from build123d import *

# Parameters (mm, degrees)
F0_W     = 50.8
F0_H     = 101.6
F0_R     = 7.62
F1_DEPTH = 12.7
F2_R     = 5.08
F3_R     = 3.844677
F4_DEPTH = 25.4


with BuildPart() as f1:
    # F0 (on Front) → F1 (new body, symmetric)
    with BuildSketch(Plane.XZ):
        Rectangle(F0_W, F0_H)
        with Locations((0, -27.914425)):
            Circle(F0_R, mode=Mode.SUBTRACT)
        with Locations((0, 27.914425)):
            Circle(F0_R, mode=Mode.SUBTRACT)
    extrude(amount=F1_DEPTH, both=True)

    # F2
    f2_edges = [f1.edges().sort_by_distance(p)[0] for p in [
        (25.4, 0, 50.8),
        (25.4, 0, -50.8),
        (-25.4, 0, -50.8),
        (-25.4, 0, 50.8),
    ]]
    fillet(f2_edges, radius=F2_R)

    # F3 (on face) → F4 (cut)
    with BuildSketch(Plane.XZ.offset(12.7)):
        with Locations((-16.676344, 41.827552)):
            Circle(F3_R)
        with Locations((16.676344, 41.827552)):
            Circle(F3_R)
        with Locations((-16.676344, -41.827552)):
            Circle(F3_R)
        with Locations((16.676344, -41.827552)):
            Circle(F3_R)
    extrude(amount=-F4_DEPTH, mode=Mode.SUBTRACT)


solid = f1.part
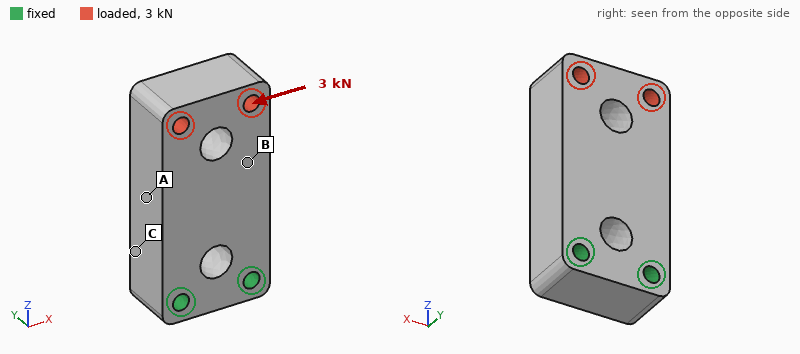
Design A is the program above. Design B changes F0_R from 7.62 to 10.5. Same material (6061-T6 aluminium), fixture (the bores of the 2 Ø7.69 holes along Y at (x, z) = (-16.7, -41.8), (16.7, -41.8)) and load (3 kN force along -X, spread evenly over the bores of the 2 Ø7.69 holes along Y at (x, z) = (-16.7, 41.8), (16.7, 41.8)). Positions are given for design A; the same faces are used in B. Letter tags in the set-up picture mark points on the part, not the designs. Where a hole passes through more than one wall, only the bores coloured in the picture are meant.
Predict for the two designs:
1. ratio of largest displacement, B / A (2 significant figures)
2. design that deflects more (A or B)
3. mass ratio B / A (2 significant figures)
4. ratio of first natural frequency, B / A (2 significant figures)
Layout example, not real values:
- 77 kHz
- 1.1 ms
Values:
- 1.1
- B
- 0.93
- 0.97
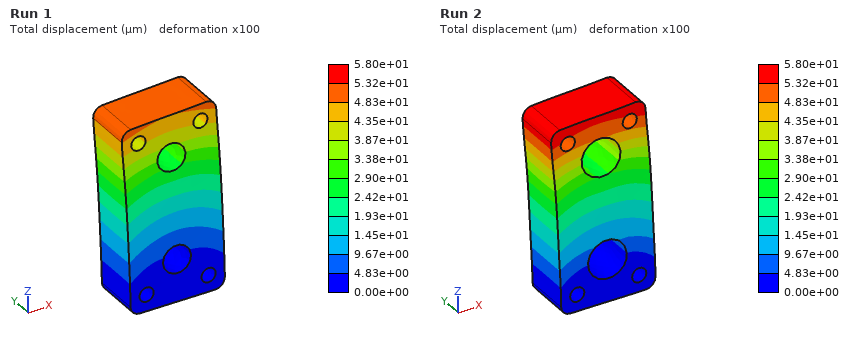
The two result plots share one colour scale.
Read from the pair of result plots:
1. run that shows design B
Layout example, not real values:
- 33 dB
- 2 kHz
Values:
- Run 2
